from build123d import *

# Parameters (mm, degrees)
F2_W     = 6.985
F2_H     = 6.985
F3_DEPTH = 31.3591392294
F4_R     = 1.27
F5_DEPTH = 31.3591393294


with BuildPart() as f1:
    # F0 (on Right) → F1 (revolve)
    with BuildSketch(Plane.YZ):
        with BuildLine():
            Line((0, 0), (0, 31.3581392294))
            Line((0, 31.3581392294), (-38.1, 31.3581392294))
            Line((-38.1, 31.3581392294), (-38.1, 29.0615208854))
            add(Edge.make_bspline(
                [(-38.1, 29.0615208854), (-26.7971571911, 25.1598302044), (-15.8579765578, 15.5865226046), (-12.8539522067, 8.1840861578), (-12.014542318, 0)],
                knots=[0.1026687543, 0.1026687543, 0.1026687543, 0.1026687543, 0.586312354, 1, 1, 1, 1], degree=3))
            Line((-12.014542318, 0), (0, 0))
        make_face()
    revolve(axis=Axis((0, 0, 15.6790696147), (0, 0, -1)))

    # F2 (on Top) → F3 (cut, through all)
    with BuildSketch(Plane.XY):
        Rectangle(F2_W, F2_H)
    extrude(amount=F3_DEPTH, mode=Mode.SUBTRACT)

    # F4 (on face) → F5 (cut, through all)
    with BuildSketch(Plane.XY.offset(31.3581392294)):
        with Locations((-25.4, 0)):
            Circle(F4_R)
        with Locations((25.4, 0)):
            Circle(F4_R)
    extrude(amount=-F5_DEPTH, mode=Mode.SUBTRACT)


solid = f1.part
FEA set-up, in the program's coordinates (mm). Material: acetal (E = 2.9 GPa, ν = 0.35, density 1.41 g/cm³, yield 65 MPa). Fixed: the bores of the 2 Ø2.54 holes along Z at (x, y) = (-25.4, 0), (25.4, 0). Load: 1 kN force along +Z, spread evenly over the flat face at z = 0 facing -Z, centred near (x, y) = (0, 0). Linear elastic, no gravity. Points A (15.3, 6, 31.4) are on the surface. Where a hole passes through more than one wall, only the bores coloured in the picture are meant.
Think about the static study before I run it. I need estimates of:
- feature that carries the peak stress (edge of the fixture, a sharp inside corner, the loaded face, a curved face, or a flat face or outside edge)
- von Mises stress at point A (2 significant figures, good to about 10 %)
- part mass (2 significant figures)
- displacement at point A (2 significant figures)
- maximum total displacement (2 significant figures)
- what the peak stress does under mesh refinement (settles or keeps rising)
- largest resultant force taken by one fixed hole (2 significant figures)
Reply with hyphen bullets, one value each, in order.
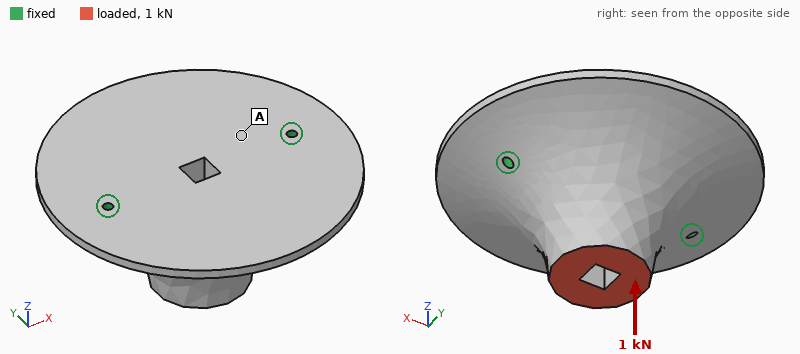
- edge of the fixture
- 2.1 MPa
- 67 g
- 47 µm
- 83 µm
- keeps rising
- 580 N
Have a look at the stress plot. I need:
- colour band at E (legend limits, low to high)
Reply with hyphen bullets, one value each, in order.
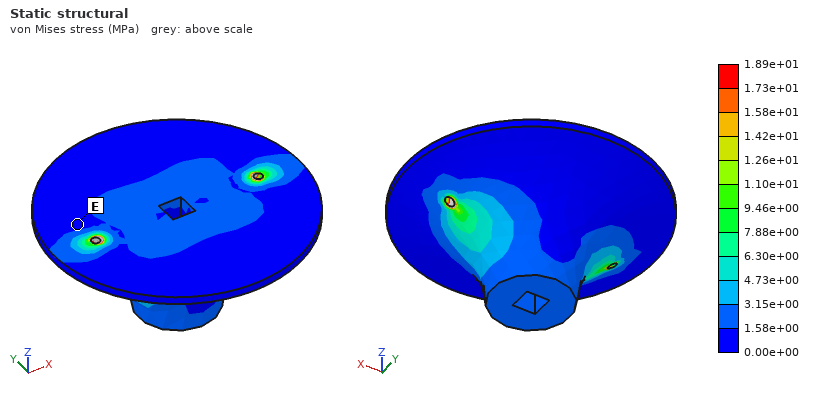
- 0.00e+00 to 1.58e+00 MPa
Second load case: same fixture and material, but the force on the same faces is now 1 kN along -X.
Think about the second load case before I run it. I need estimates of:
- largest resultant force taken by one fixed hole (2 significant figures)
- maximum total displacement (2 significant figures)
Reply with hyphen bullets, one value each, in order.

- 740 N
- 0.12 mm
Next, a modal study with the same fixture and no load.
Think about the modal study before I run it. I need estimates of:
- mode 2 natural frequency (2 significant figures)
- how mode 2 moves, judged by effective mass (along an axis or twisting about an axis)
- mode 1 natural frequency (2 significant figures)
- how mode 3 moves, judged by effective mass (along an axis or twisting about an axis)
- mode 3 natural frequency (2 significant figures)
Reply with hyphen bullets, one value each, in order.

- 2500 Hz
- along Z
- 1000 Hz
- twisting about Y
- 4100 Hz
